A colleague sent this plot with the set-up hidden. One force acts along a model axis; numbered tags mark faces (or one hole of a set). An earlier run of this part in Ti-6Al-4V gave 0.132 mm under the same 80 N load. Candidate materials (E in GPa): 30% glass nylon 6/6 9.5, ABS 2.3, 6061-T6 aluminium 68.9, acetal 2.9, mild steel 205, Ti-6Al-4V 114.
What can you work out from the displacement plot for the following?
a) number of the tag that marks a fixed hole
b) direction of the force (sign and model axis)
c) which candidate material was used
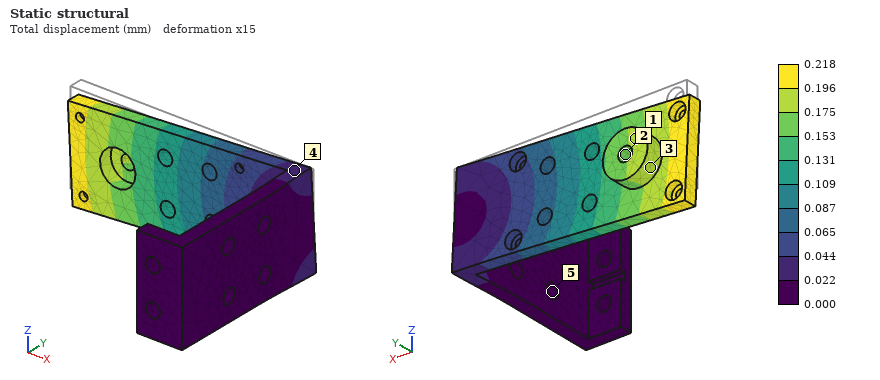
5
-Z
6061-T6 aluminium
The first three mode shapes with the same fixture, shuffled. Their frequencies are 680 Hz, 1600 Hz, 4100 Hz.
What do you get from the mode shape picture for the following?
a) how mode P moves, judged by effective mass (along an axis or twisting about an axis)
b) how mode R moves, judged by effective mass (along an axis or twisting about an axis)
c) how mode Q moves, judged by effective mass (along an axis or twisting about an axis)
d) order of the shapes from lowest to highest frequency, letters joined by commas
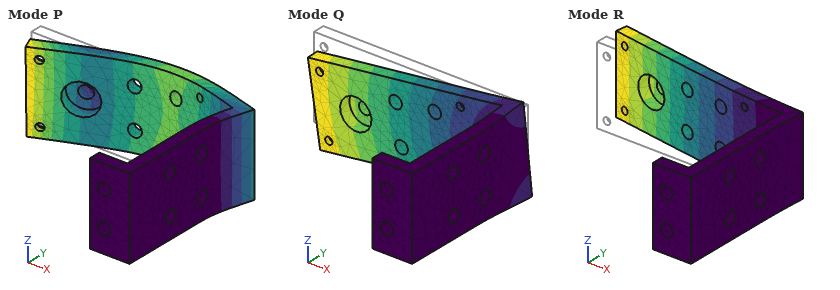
along X
along Y
along Z
R, Q, P
